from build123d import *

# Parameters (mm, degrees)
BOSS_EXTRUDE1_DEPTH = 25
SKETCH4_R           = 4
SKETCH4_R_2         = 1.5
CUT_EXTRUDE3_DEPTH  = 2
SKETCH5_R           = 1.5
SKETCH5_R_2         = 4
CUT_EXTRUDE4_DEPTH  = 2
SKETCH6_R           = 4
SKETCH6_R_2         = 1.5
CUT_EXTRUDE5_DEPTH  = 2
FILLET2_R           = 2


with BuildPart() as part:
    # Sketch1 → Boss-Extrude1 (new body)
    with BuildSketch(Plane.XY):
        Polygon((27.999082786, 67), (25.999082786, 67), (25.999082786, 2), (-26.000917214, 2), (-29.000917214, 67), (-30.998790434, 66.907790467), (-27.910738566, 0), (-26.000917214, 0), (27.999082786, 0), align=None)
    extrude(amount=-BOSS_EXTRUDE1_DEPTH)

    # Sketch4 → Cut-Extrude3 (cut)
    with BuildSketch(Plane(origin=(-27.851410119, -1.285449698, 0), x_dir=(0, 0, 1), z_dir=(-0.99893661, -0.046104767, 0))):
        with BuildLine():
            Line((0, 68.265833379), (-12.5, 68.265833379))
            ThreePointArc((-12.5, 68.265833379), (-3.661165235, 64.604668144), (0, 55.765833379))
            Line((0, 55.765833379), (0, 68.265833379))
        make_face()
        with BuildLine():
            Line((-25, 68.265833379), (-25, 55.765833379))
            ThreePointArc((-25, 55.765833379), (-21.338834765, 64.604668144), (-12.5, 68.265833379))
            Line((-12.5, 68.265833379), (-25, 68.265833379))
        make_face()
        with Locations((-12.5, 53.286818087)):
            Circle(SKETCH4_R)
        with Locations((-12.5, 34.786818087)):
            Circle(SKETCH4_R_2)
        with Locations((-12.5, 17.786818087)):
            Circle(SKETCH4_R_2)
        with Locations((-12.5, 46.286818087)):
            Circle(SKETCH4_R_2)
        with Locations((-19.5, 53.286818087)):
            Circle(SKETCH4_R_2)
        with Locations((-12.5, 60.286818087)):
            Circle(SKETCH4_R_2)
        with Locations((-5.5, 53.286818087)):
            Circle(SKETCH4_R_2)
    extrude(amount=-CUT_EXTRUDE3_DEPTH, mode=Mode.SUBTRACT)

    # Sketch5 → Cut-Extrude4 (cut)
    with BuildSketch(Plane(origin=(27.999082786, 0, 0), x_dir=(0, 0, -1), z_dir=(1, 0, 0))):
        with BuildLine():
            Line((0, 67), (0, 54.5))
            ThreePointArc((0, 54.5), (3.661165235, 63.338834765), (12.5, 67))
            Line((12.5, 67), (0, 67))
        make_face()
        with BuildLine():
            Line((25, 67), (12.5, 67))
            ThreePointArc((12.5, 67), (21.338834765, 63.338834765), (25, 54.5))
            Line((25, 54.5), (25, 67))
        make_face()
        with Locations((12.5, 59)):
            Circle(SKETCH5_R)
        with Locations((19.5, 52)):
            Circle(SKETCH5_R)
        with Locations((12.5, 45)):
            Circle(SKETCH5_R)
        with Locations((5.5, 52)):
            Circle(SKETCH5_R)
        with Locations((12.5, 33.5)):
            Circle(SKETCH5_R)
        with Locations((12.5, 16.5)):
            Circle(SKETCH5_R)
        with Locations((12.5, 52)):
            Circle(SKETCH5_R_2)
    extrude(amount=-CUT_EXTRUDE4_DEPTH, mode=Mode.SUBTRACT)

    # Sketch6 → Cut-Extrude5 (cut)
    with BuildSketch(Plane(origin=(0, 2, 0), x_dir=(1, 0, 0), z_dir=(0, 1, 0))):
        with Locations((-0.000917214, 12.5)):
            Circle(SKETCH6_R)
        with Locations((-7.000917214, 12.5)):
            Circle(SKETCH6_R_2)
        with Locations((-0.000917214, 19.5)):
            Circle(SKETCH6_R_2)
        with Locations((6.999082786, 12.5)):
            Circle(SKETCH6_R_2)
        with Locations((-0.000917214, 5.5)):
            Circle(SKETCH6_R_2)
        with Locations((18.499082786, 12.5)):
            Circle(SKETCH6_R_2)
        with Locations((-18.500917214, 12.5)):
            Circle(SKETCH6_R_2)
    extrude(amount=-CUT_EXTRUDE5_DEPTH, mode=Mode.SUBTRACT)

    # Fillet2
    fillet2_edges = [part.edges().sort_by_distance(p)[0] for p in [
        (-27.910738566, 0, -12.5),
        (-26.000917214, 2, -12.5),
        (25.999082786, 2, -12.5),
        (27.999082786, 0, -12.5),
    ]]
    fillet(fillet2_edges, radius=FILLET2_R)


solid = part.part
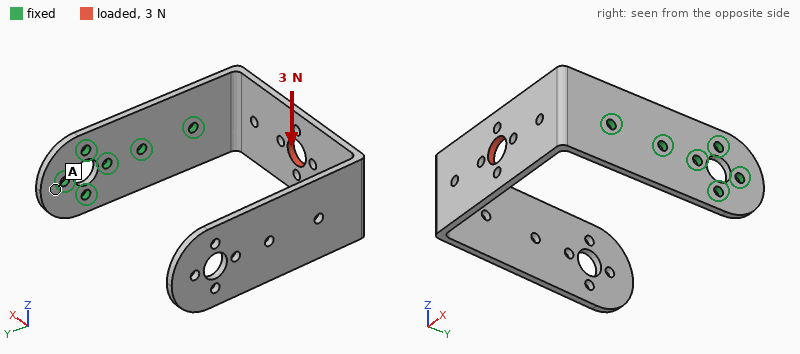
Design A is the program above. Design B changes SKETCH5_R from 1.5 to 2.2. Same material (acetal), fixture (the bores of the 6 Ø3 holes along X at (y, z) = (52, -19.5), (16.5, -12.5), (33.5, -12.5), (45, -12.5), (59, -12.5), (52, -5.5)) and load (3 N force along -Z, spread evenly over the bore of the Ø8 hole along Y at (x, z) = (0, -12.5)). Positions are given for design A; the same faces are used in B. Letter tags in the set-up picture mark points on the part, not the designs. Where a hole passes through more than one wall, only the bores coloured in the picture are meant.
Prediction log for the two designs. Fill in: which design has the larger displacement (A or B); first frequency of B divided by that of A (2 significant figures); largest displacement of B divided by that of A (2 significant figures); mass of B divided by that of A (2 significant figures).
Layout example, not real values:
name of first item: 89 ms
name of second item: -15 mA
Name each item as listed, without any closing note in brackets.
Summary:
which design has the larger displacement: A
first frequency of B divided by that of A: 1.0
largest displacement of B divided by that of A: 0.90
mass of B divided by that of A: 0.99
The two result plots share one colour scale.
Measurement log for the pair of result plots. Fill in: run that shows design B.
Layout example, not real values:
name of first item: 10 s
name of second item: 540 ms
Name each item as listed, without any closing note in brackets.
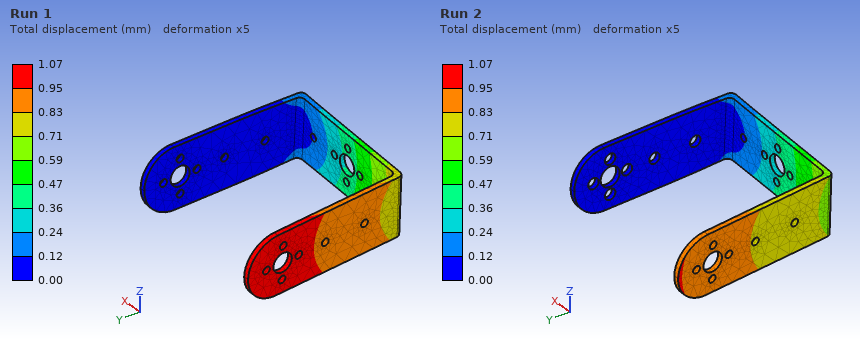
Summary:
run that shows design B: Run 2
